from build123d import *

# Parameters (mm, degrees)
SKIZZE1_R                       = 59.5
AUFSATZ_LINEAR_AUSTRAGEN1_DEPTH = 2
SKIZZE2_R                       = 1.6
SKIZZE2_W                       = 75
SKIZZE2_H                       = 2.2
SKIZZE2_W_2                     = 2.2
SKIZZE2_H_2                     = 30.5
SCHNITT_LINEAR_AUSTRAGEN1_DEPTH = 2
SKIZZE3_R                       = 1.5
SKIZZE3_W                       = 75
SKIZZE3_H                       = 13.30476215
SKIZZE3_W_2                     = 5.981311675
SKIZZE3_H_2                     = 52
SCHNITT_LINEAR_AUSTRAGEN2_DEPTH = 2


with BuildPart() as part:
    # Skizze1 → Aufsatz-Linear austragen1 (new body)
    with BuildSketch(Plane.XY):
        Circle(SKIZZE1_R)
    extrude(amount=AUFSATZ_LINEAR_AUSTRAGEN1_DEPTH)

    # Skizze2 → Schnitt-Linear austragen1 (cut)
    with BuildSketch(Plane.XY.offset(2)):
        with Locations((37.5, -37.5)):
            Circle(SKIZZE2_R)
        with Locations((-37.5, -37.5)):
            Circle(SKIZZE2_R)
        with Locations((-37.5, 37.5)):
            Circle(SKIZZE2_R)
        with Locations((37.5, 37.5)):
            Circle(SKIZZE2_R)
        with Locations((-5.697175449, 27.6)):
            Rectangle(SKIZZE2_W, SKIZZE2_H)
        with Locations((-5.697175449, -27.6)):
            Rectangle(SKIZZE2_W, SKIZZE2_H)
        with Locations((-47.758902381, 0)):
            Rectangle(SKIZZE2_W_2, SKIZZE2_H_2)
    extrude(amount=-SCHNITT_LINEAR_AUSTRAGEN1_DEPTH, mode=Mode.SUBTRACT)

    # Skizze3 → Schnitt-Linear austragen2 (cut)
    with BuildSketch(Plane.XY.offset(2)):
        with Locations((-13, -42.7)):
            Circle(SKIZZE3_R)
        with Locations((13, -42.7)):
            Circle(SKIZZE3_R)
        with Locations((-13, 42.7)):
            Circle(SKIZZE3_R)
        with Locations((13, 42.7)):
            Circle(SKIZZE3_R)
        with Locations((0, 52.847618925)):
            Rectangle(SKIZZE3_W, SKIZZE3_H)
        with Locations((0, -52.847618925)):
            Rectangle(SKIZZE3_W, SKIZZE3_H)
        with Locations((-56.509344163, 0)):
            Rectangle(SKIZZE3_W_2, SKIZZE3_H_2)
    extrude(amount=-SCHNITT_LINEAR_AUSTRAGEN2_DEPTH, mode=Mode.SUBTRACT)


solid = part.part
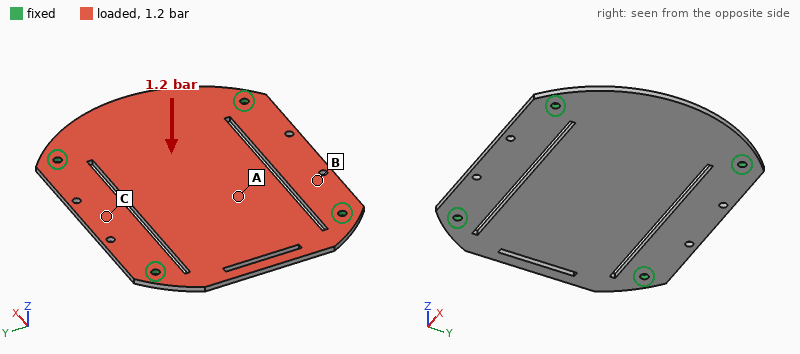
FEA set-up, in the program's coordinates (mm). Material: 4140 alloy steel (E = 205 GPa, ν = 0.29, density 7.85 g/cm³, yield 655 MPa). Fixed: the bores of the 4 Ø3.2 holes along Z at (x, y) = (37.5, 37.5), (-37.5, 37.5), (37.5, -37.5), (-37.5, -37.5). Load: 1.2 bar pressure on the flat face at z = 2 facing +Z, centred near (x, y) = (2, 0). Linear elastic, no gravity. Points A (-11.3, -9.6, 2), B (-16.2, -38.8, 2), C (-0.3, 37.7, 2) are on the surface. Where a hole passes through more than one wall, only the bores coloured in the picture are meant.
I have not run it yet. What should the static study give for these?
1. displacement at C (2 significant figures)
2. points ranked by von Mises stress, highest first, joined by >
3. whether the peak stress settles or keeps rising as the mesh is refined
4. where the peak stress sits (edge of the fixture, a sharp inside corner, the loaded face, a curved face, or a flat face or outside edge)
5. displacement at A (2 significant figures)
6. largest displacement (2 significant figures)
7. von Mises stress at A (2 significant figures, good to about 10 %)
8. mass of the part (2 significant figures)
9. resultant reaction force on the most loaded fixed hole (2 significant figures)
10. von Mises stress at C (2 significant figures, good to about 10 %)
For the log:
0.070 mm
A > C > B
keeps rising
edge of the fixture
0.31 mm
0.32 mm
67 MPa
140 g
300 N
39 MPa
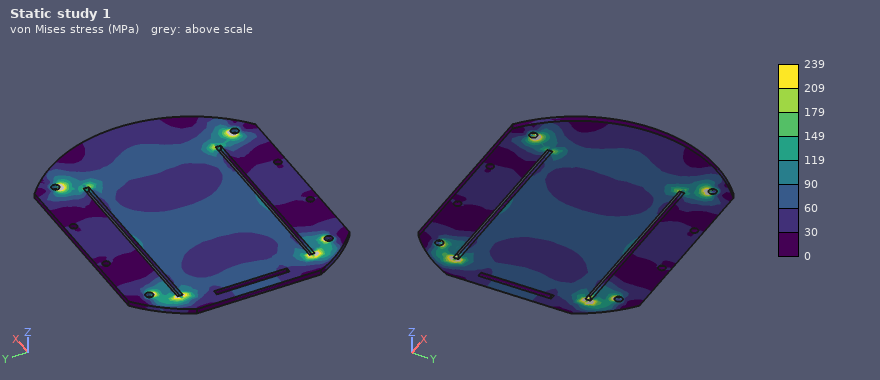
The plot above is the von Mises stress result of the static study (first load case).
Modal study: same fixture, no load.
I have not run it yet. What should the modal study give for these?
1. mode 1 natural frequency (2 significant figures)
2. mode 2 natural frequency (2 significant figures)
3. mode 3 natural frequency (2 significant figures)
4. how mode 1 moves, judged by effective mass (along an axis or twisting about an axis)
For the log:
890 Hz
1500 Hz
1700 Hz
along Z
